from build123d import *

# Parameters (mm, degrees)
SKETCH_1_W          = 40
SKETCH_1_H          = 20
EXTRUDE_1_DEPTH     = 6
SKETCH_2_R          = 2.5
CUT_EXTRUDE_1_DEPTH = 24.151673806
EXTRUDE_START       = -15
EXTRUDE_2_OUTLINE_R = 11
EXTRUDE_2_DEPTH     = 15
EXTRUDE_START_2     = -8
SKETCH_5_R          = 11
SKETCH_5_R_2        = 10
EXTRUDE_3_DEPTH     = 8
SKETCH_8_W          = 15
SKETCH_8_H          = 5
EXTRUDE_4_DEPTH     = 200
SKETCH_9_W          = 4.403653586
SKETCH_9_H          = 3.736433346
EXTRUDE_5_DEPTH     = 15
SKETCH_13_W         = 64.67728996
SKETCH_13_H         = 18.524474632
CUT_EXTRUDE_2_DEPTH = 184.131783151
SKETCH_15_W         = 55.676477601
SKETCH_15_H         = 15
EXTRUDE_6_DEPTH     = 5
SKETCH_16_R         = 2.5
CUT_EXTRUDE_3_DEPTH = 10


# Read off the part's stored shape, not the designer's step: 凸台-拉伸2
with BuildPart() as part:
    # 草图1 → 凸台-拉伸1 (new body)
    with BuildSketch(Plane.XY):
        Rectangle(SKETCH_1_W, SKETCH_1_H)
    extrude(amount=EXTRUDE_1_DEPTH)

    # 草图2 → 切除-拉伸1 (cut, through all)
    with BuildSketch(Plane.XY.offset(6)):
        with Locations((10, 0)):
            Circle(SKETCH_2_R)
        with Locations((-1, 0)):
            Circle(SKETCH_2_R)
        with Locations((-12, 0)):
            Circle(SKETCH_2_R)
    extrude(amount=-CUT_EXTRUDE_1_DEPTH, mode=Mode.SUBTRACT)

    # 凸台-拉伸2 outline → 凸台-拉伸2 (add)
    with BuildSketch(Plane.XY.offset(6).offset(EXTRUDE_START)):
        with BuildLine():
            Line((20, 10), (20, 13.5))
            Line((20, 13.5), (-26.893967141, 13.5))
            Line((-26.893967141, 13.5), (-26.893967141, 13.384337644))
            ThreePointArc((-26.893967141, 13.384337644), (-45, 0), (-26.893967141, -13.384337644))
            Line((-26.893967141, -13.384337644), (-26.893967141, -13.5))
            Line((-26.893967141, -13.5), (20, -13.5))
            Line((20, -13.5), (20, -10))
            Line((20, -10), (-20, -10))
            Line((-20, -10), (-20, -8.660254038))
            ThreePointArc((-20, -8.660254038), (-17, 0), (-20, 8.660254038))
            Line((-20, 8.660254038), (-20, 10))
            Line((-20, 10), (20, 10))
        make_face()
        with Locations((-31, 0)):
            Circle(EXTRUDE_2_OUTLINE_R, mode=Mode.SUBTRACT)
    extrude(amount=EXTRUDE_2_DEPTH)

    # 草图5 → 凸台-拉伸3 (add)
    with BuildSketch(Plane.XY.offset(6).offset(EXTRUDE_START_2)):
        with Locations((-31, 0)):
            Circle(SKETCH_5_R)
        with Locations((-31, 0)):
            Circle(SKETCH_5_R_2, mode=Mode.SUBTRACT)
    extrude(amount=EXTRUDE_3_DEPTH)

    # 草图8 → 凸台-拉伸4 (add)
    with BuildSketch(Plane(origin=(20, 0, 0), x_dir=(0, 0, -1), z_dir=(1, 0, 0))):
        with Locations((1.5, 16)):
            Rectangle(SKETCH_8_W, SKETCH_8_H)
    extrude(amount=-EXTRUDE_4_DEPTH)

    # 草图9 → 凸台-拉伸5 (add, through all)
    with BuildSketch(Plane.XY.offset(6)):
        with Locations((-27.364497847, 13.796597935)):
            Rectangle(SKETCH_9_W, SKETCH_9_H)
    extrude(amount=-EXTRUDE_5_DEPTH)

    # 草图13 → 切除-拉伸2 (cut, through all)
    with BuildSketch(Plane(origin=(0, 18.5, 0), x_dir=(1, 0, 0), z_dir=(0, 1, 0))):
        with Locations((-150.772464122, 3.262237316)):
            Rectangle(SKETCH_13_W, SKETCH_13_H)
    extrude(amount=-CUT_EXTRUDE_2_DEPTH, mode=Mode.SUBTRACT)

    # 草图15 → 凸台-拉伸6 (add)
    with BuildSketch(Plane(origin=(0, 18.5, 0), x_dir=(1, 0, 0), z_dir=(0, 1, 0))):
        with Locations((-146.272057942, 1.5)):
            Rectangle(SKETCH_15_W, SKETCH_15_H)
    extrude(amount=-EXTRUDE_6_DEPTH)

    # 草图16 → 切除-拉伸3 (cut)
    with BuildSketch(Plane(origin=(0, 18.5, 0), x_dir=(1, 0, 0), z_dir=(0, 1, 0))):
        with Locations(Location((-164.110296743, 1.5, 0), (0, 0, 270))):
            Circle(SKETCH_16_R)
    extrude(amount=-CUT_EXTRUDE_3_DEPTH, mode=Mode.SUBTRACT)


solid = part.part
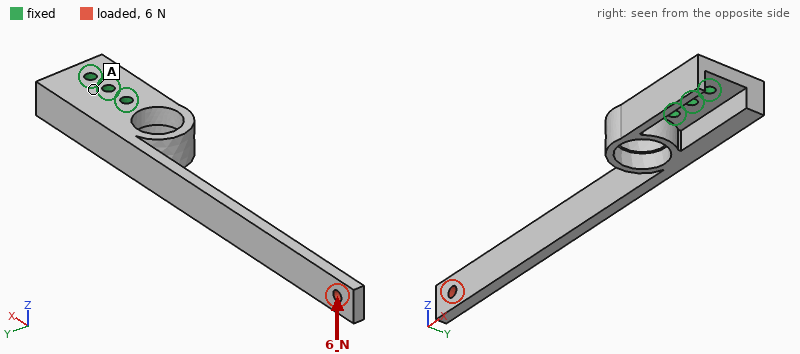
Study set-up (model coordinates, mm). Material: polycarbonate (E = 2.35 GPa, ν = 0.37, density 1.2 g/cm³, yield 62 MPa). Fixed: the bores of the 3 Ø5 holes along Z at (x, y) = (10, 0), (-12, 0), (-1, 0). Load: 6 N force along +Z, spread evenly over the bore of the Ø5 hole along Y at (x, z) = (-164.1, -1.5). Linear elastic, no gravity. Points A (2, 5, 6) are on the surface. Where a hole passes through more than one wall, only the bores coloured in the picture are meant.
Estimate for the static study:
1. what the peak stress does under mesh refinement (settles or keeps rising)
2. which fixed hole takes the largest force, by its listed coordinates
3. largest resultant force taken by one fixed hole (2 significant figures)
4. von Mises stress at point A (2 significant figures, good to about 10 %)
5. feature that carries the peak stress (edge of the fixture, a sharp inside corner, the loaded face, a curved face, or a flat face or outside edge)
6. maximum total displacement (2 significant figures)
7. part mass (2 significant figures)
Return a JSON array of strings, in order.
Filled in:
["keeps rising", "(-12, 0)", "40 N", "0.45 MPa", "edge of the fixture", "2.2 mm", "33 g"]
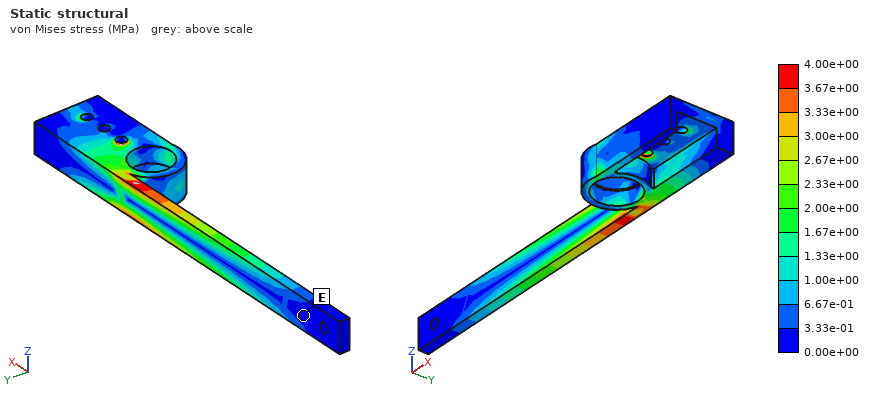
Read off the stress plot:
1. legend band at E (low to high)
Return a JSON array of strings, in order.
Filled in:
["0.00e+00 to 3.33e-01 MPa"]
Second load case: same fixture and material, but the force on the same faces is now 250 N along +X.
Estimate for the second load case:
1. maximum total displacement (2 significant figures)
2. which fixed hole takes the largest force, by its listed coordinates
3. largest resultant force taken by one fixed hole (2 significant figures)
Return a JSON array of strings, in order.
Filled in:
["0.81 mm", "(-12, 0)", "190 N"]
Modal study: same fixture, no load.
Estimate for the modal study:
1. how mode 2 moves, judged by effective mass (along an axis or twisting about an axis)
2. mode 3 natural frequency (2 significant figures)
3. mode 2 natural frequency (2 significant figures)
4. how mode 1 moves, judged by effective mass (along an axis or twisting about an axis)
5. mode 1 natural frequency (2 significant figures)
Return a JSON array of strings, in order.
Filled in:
["along Z", "340 Hz", "140 Hz", "along Y", "56 Hz"]
